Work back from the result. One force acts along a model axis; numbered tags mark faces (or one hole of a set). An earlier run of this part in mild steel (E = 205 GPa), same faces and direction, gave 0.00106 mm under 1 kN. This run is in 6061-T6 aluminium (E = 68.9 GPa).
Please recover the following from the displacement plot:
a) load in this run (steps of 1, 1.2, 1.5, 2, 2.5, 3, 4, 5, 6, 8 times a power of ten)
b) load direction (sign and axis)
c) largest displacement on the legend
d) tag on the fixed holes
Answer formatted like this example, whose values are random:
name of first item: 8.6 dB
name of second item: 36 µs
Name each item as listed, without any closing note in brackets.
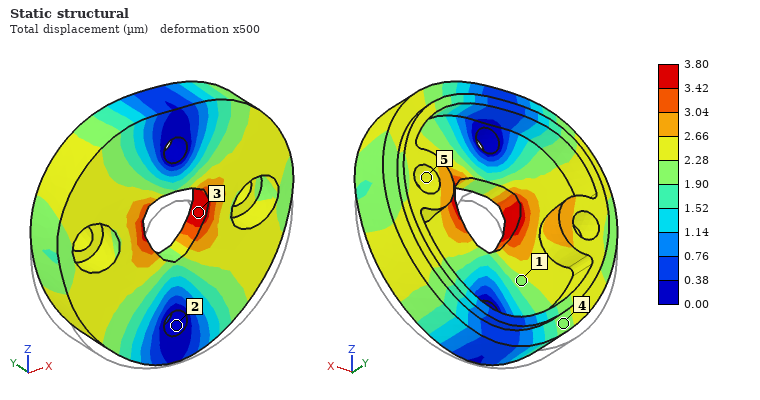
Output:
load in this run: 1.2 kN
load direction: +Z
largest displacement on the legend: 3.80 µm
tag on the fixed holes: 2
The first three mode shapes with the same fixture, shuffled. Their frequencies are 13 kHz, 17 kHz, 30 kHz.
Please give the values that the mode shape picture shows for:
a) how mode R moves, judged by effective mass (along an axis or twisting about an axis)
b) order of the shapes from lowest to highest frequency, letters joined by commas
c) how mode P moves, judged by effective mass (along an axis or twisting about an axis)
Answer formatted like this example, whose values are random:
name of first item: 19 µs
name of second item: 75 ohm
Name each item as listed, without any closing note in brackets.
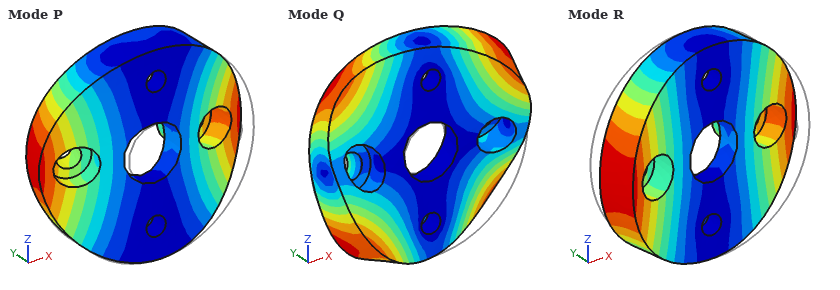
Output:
how mode R moves, judged by effective mass: twisting about Z
order of the shapes from lowest to highest frequency, letters joined by commas: R, P, Q
how mode P moves, judged by effective mass: along Y
